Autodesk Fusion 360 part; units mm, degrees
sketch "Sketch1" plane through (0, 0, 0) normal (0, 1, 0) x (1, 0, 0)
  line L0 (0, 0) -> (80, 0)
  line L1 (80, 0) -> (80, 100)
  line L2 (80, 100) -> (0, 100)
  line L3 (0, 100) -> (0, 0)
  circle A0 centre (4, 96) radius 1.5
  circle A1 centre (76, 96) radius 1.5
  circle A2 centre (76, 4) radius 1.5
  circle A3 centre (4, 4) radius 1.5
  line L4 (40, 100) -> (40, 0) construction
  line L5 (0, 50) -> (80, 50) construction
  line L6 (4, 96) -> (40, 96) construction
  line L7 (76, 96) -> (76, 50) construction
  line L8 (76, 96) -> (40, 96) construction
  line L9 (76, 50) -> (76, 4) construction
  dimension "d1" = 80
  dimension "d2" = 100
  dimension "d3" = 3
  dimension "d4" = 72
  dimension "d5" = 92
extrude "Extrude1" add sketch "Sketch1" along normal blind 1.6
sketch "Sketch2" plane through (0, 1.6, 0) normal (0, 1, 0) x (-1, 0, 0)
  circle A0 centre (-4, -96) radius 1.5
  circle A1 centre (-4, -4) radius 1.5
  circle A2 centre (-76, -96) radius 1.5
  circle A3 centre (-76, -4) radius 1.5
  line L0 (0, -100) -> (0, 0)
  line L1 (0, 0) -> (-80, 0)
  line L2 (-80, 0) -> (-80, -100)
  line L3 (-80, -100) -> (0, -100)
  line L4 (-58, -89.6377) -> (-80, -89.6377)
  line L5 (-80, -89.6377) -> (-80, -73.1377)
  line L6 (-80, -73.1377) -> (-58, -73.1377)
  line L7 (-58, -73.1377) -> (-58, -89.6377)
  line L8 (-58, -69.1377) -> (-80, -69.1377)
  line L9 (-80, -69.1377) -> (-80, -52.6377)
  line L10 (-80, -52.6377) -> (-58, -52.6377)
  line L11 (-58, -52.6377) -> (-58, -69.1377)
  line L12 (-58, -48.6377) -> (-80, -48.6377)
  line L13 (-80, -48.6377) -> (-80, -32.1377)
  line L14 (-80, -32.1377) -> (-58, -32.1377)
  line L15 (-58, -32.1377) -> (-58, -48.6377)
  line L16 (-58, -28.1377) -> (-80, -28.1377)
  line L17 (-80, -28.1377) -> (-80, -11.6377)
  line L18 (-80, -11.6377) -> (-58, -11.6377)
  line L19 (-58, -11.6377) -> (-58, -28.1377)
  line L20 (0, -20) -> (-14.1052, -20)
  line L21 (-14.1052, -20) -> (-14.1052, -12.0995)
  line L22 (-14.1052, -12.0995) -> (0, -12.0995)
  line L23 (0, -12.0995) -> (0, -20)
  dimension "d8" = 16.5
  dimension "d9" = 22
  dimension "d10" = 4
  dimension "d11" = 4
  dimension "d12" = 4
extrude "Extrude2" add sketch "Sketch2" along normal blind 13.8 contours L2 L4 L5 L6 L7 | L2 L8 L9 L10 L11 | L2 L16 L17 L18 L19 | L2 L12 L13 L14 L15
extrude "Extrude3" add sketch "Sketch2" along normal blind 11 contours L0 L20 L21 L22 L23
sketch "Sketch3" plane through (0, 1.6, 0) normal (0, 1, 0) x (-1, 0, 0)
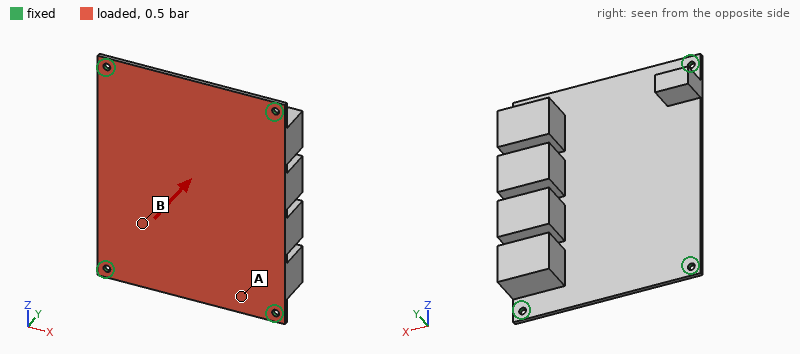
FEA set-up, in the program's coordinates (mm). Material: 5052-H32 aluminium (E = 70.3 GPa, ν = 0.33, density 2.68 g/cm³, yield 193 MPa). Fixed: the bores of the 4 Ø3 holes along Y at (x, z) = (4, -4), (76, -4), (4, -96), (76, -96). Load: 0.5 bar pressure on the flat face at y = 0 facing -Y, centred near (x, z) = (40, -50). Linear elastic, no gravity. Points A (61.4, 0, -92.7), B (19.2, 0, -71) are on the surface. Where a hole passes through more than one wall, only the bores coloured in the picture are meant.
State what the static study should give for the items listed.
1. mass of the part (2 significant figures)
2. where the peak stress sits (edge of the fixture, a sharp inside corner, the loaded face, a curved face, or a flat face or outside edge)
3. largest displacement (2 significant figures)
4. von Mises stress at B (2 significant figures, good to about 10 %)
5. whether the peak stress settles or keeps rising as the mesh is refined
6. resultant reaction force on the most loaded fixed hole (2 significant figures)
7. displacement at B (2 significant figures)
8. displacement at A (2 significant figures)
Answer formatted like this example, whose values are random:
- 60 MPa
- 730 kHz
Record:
- 91 g
- edge of the fixture
- 0.61 mm
- 31 MPa
- keeps rising
- 130 N
- 0.44 mm
- 0.13 mm
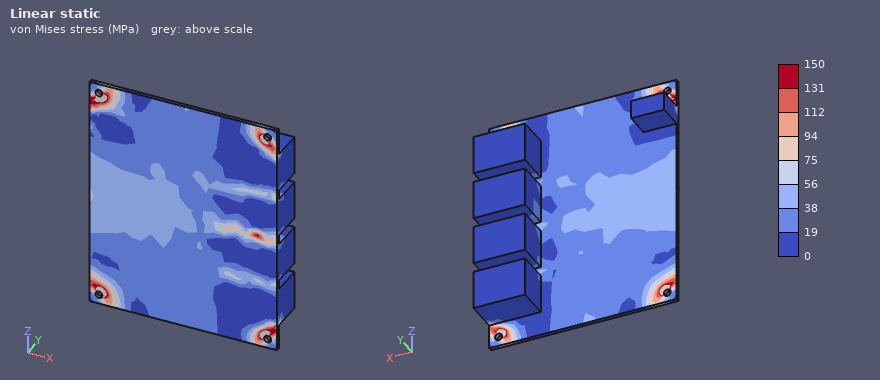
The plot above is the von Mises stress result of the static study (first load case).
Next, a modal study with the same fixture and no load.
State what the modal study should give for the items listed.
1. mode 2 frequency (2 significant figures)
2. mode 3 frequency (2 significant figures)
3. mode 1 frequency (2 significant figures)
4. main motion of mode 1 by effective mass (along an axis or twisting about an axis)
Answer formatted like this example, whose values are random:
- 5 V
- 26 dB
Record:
- 990 Hz
- 1400 Hz
- 540 Hz
- along Y
